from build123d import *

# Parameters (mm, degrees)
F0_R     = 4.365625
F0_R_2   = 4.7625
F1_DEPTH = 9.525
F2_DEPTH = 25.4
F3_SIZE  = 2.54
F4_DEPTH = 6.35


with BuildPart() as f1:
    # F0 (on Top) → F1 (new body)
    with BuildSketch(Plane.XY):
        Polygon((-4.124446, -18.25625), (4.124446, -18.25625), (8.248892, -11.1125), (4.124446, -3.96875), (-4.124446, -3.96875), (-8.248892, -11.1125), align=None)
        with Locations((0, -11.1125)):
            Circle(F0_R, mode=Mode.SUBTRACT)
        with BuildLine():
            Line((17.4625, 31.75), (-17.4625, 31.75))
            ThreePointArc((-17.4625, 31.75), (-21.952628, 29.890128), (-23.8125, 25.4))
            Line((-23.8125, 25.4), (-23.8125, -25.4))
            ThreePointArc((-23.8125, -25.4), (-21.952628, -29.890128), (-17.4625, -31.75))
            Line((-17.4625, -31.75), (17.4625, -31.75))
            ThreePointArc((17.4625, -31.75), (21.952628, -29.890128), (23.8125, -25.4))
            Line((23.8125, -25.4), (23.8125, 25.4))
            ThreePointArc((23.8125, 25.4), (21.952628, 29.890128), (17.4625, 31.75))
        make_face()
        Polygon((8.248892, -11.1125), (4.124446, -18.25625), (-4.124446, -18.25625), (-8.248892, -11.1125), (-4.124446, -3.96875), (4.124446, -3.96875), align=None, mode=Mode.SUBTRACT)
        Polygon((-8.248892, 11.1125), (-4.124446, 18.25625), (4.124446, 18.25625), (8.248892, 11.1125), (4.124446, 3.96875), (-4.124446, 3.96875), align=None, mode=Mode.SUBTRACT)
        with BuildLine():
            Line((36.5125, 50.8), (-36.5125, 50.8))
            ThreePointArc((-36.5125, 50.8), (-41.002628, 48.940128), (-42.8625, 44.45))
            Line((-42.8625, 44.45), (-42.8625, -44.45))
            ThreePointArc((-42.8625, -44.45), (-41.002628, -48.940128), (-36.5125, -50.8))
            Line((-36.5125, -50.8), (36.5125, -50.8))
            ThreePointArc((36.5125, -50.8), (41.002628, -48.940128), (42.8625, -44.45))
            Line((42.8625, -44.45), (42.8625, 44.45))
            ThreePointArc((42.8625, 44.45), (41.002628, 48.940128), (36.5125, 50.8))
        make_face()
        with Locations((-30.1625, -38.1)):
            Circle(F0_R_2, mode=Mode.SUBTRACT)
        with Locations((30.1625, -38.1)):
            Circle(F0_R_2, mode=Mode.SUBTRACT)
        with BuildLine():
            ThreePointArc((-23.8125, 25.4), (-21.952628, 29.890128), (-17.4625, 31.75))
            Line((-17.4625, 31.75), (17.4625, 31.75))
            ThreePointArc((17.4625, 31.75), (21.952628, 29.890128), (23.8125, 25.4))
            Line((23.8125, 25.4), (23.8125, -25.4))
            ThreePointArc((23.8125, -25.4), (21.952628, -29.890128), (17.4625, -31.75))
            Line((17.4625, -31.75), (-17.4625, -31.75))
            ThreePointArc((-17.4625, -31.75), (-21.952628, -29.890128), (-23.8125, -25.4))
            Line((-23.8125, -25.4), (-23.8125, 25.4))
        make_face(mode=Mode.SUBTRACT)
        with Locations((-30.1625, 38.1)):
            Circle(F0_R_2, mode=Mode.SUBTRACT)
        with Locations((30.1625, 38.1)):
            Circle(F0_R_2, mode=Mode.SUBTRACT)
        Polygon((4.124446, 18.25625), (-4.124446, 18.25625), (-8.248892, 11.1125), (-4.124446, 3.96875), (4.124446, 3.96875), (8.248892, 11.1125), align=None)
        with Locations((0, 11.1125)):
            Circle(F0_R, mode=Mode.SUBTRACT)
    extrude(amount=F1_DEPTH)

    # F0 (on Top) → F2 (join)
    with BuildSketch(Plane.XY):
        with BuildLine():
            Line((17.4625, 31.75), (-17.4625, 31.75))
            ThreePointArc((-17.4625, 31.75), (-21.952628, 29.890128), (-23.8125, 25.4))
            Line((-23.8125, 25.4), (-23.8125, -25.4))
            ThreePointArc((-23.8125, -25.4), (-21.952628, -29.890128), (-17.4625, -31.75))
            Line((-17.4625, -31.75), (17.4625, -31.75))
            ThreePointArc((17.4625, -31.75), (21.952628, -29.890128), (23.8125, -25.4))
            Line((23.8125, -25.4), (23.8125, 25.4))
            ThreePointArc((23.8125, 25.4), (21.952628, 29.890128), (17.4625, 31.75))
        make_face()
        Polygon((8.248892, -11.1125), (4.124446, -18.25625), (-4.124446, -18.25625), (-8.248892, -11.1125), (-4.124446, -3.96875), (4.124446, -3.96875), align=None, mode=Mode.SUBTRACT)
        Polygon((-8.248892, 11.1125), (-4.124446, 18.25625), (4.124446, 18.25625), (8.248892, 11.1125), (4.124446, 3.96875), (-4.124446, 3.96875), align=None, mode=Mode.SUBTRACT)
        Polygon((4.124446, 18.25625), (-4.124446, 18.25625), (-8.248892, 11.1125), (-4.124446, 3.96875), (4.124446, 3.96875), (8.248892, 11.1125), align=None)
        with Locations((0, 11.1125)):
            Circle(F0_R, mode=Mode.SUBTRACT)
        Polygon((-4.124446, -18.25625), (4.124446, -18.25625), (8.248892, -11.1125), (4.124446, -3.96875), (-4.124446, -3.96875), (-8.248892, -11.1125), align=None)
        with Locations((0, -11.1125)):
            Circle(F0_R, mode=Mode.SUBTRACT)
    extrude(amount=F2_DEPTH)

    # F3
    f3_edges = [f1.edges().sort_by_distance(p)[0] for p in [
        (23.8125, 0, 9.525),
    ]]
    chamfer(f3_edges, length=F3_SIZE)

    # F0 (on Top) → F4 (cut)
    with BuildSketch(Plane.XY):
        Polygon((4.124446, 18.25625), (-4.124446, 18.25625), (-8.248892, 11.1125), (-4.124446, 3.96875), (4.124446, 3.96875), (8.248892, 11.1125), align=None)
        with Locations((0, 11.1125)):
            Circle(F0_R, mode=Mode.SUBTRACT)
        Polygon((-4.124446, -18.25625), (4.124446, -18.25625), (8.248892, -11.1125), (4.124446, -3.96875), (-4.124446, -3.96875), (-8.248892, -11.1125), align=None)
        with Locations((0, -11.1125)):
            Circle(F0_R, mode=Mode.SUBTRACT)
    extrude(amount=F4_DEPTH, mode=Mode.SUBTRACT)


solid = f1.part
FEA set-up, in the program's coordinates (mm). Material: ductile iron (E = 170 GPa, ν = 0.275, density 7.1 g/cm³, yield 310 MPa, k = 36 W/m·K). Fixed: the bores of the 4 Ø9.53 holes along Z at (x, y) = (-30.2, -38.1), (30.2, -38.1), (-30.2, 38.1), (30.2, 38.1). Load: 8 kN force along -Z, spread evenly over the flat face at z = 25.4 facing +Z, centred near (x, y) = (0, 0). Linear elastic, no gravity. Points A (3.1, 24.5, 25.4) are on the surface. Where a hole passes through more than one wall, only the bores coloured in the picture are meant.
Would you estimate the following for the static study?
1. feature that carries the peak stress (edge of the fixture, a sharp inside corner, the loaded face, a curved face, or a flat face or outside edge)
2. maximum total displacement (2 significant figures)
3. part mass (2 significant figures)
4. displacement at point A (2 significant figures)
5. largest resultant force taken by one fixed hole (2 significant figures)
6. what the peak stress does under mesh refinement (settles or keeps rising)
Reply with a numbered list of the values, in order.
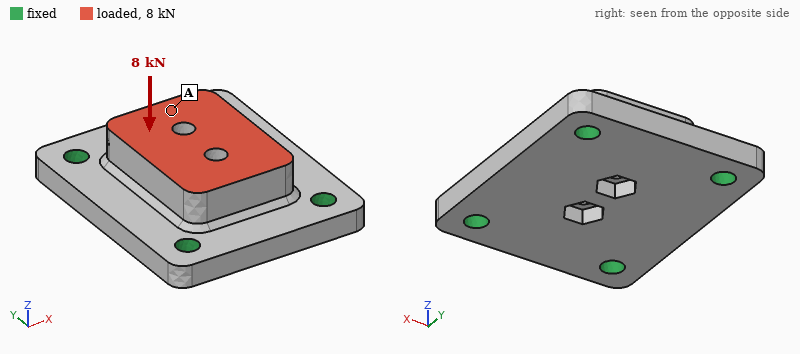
1. edge of the fixture
2. 5.8 µm
3. 880 g
4. 4.6 µm
5. 2.3 kN
6. keeps rising
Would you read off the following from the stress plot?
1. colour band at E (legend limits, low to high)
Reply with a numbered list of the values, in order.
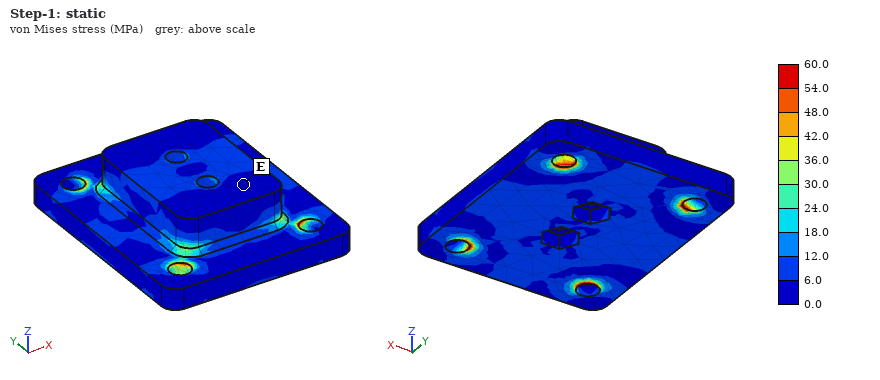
1. 0.0 to 6.0 MPa
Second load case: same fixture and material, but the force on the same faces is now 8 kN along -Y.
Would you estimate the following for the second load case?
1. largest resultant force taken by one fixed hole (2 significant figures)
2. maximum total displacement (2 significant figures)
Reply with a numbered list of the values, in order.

1. 2.5 kN
2. 4.3 µm
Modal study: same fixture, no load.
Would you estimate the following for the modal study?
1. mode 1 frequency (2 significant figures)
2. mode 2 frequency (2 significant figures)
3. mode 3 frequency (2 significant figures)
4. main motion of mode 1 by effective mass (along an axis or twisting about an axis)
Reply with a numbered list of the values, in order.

1. 8000 Hz
2. 10 kHz
3. 13 kHz
4. along Z
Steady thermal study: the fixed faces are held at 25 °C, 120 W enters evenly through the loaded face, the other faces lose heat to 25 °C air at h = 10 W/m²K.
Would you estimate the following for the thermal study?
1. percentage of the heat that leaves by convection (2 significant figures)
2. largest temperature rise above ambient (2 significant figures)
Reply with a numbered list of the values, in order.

1. 5.6 %
2. 69 K
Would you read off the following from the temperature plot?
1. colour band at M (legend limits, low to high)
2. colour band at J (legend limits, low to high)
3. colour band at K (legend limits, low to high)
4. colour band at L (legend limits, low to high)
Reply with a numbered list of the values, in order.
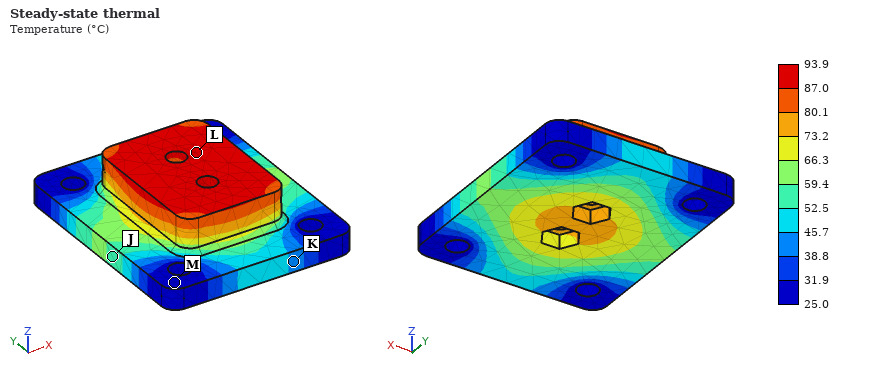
1. 25.0 to 31.9 °C
2. 52.5 to 59.4 °C
3. 38.8 to 45.7 °C
4. 87.0 to 93.9 °C
